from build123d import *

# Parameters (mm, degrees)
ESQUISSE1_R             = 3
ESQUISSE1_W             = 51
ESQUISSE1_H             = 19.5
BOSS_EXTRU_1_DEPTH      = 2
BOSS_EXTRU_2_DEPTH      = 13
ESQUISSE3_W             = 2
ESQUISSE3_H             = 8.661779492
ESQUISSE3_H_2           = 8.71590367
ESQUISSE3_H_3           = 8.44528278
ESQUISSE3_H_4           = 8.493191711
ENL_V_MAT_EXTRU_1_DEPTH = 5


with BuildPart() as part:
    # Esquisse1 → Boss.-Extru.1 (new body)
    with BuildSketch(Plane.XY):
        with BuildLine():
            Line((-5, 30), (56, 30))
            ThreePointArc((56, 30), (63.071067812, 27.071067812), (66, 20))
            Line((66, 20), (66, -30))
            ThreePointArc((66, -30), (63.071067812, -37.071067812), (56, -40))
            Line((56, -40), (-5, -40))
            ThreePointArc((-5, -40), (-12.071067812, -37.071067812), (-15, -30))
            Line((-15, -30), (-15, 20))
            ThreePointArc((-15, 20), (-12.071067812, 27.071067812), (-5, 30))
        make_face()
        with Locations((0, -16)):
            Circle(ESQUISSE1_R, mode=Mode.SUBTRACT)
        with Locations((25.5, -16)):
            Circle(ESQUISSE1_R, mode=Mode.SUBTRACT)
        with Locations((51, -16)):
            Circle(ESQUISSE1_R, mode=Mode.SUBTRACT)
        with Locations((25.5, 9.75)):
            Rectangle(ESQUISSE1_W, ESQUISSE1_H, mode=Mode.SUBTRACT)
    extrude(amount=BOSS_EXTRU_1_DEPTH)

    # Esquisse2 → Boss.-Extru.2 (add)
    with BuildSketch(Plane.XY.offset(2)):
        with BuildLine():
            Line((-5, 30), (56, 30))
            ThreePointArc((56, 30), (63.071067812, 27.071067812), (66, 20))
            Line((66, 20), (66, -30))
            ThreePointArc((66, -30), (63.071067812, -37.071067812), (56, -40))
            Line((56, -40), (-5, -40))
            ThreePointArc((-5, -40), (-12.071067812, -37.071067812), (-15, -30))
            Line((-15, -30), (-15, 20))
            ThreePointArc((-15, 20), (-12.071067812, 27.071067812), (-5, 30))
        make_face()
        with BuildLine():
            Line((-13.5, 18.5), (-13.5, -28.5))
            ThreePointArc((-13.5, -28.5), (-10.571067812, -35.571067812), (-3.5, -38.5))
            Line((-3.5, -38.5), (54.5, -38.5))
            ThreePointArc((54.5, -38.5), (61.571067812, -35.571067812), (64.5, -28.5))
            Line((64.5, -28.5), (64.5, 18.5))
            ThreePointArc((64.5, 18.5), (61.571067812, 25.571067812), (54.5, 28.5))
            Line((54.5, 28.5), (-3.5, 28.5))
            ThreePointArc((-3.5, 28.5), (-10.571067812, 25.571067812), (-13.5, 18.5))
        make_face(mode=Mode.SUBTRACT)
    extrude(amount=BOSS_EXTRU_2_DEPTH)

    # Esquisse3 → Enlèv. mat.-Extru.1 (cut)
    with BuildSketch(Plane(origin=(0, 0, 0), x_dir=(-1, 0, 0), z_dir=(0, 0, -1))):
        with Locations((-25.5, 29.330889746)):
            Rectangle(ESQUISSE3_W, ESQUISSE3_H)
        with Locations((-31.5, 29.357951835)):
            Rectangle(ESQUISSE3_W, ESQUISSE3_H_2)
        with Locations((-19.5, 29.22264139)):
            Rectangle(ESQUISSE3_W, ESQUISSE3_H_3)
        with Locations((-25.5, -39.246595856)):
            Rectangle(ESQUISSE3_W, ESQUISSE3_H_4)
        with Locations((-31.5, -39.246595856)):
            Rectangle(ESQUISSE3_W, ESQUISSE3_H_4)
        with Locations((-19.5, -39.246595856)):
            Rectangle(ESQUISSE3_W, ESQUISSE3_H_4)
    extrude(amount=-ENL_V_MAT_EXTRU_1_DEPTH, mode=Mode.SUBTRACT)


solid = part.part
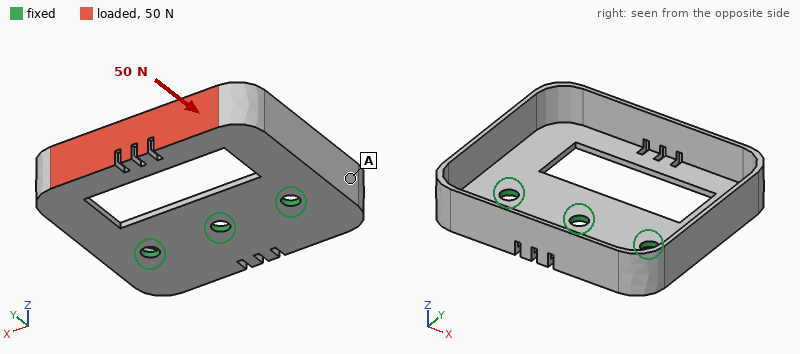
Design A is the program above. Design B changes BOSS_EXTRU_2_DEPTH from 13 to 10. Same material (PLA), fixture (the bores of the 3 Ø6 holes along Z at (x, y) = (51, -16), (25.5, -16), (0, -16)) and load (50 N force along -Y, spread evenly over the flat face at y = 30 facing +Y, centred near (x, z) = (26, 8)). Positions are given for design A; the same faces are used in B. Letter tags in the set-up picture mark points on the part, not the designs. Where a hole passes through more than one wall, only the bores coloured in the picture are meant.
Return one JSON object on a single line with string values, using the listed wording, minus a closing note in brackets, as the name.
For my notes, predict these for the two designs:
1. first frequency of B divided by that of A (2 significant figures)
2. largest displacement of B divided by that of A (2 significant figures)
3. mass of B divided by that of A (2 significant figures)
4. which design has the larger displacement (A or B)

{"first frequency of B divided by that of A": "1.0", "largest displacement of B divided by that of A": "0.82", "mass of B divided by that of A": "0.91", "which design has the larger displacement": "A"}
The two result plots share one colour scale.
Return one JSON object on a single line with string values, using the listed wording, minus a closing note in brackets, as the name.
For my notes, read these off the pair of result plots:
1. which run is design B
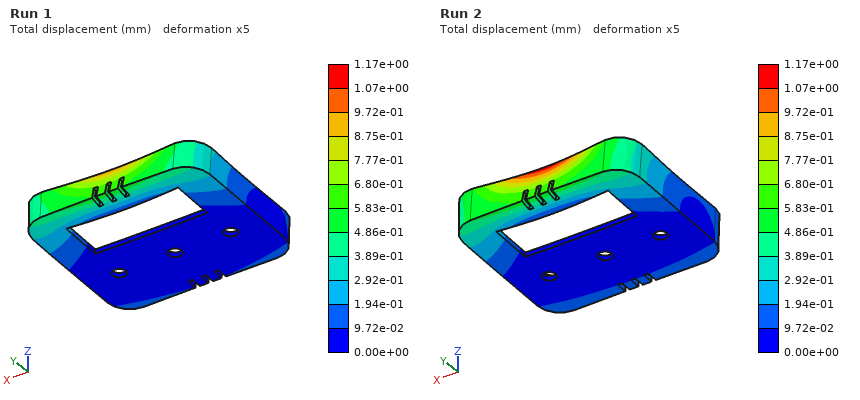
{"which run is design B": "Run 1"}
